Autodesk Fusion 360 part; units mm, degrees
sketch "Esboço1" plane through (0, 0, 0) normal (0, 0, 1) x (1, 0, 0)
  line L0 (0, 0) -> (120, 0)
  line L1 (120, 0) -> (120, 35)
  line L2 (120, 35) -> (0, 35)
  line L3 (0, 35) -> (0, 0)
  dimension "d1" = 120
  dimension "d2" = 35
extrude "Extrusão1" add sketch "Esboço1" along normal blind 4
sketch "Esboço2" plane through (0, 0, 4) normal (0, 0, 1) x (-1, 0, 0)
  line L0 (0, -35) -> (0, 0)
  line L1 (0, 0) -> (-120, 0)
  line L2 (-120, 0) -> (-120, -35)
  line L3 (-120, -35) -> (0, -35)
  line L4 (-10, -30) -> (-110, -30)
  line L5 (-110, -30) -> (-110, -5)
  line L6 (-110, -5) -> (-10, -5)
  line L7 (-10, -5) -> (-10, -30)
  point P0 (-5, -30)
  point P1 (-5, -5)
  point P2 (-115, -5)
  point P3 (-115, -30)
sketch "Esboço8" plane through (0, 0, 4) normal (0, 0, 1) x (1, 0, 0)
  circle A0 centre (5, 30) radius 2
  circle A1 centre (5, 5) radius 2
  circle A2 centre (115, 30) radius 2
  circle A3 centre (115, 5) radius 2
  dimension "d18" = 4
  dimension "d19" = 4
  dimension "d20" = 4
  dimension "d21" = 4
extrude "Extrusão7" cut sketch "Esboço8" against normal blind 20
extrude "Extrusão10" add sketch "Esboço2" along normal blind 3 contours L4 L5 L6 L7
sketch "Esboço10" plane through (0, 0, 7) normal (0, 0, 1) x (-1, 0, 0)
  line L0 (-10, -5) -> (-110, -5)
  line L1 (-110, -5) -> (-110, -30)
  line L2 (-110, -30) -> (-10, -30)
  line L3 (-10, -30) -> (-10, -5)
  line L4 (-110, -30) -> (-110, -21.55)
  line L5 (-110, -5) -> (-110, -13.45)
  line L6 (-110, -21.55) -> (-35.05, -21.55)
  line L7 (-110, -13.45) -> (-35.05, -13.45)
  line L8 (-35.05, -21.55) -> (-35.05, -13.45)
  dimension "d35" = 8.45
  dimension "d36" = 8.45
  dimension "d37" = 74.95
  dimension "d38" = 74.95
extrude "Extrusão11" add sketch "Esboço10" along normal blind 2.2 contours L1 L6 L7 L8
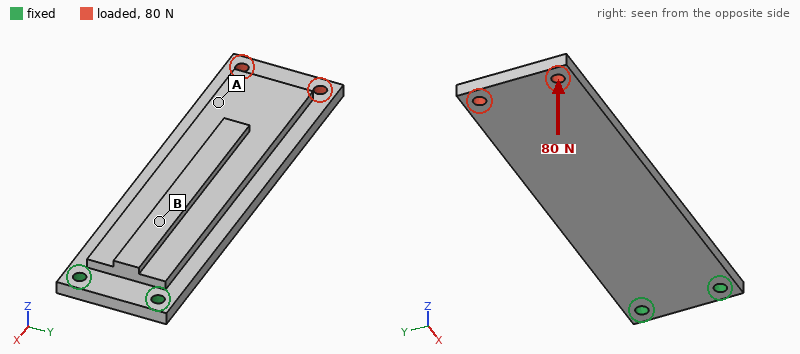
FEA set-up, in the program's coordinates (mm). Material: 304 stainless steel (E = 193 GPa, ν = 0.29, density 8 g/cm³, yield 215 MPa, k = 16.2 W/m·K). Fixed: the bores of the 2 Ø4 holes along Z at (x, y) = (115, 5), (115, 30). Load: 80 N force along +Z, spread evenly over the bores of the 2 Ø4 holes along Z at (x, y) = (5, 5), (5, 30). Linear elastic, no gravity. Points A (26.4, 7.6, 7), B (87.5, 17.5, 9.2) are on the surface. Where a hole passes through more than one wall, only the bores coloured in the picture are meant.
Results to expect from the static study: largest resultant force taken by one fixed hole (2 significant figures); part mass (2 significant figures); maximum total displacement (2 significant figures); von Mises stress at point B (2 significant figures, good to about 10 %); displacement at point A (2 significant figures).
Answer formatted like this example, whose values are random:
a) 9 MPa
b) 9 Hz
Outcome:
a) 58 N
b) 200 g
c) 0.34 mm
d) 31 MPa
e) 0.24 mm
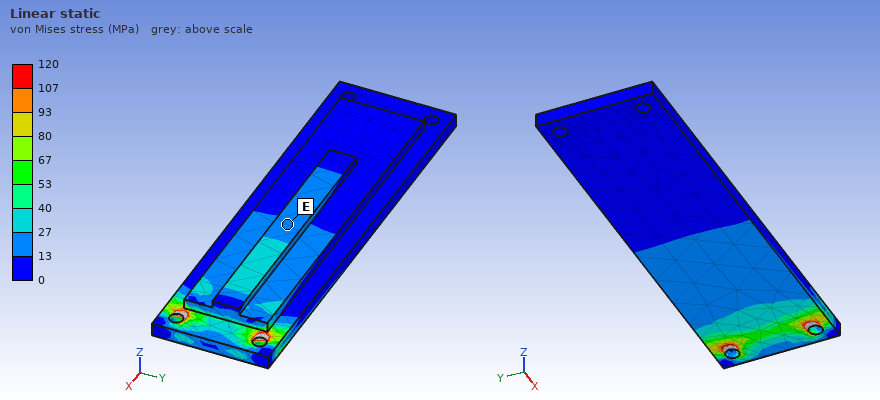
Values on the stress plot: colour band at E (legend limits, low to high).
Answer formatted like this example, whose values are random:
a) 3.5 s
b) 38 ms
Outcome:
a) 13 to 27 MPa
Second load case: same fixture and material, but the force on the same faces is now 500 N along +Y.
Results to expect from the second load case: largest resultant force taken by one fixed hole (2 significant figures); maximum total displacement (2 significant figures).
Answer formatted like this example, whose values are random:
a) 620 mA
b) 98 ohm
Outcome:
a) 2.1 kN
b) 81 µm
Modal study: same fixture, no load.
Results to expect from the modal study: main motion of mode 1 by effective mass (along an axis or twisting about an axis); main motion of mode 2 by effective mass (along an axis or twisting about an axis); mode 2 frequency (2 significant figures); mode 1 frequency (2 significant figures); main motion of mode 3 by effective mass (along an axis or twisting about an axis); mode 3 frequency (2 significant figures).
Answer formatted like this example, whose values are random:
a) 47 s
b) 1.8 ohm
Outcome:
a) along Z
b) along Y
c) 1800 Hz
d) 330 Hz
e) along Z
f) 2500 Hz
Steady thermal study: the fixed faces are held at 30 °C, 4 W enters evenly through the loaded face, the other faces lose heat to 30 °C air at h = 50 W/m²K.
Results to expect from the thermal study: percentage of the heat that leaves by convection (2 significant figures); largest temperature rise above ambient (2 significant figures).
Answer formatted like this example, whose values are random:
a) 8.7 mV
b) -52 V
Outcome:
a) 97 %
b) 37 K
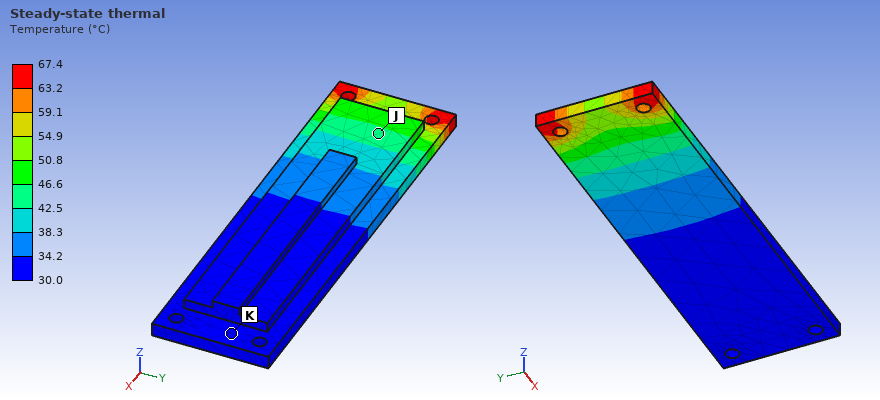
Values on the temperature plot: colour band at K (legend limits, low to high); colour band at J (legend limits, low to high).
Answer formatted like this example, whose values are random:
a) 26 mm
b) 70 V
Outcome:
a) 30.0 to 34.2 °C
b) 42.5 to 46.6 °C
